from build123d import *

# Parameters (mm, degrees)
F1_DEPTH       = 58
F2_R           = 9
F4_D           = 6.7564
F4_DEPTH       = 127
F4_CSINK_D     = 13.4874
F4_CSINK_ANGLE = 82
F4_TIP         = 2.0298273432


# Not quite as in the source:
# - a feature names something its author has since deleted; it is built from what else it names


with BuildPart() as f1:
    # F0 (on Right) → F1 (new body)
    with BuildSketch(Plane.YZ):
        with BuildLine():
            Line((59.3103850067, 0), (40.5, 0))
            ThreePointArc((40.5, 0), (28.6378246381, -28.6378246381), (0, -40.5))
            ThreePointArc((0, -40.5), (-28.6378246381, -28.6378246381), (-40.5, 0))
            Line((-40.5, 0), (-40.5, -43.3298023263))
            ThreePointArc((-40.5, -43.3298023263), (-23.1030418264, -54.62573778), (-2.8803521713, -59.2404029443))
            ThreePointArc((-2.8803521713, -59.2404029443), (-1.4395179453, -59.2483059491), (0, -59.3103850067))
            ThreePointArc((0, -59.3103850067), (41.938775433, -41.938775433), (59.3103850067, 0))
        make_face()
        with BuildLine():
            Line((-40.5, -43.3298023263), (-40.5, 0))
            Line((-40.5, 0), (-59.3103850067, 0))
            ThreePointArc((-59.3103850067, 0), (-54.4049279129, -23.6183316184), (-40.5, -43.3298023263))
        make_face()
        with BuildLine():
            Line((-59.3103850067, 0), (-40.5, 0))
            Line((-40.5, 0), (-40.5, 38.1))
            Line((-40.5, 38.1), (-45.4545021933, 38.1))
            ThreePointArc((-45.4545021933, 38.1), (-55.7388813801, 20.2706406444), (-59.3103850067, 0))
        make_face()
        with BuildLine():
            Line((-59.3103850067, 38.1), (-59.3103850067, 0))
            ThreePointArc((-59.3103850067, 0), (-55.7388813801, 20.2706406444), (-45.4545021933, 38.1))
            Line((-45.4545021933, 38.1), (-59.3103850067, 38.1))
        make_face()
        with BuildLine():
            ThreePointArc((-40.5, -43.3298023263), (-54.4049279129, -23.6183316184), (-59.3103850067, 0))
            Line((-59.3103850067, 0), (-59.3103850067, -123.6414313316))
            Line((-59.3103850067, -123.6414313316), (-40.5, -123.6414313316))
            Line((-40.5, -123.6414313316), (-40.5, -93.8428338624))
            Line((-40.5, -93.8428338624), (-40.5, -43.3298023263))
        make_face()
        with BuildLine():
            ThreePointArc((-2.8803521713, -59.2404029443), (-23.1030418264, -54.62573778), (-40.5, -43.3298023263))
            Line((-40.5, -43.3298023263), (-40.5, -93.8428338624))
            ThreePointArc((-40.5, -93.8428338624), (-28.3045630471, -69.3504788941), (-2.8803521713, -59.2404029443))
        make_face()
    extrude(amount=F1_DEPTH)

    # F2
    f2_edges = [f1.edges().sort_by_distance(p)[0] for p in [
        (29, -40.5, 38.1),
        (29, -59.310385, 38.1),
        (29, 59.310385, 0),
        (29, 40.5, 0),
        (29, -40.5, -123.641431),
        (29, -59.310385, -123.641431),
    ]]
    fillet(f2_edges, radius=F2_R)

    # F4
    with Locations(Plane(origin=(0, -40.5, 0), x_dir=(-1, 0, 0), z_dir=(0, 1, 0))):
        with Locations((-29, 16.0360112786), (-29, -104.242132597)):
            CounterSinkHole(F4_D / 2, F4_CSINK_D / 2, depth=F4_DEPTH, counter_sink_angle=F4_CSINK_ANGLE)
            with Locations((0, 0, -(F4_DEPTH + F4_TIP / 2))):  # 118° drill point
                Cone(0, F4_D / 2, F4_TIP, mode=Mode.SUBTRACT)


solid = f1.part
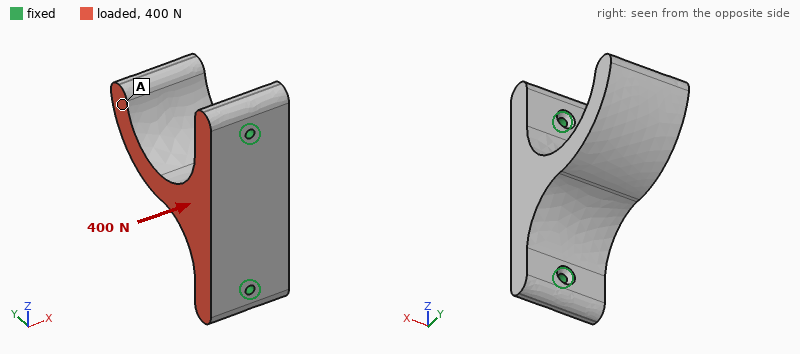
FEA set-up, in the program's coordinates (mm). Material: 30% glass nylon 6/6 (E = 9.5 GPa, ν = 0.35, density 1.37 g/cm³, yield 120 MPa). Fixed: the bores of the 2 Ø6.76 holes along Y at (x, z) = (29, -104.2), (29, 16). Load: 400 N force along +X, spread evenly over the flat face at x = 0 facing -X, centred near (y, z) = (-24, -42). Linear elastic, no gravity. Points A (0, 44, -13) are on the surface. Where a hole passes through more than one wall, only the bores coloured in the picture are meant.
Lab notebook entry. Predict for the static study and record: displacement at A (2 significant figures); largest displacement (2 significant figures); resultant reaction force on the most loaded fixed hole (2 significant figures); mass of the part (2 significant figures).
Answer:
85 µm
97 µm
210 N
460 g
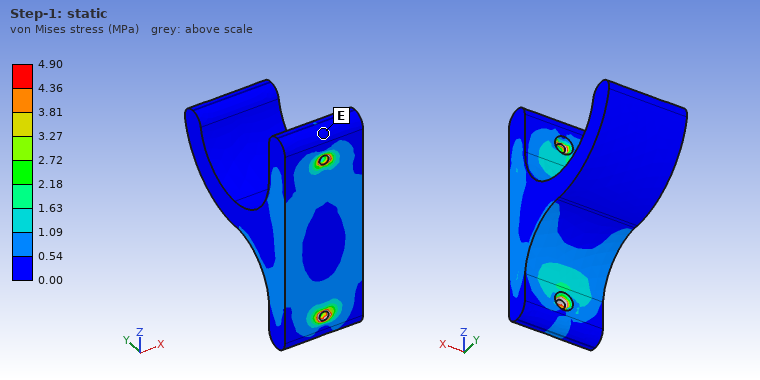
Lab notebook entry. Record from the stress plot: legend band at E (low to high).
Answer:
0.00 to 0.54 MPa
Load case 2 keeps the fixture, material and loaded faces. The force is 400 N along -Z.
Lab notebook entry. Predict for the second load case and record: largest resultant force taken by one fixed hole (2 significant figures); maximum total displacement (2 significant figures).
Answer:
250 N
55 µm
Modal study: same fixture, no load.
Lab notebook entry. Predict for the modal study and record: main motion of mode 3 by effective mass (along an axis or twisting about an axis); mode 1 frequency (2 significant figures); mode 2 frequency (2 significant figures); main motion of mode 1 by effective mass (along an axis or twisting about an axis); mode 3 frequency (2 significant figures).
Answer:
along Y
580 Hz
820 Hz
along X
1900 Hz
